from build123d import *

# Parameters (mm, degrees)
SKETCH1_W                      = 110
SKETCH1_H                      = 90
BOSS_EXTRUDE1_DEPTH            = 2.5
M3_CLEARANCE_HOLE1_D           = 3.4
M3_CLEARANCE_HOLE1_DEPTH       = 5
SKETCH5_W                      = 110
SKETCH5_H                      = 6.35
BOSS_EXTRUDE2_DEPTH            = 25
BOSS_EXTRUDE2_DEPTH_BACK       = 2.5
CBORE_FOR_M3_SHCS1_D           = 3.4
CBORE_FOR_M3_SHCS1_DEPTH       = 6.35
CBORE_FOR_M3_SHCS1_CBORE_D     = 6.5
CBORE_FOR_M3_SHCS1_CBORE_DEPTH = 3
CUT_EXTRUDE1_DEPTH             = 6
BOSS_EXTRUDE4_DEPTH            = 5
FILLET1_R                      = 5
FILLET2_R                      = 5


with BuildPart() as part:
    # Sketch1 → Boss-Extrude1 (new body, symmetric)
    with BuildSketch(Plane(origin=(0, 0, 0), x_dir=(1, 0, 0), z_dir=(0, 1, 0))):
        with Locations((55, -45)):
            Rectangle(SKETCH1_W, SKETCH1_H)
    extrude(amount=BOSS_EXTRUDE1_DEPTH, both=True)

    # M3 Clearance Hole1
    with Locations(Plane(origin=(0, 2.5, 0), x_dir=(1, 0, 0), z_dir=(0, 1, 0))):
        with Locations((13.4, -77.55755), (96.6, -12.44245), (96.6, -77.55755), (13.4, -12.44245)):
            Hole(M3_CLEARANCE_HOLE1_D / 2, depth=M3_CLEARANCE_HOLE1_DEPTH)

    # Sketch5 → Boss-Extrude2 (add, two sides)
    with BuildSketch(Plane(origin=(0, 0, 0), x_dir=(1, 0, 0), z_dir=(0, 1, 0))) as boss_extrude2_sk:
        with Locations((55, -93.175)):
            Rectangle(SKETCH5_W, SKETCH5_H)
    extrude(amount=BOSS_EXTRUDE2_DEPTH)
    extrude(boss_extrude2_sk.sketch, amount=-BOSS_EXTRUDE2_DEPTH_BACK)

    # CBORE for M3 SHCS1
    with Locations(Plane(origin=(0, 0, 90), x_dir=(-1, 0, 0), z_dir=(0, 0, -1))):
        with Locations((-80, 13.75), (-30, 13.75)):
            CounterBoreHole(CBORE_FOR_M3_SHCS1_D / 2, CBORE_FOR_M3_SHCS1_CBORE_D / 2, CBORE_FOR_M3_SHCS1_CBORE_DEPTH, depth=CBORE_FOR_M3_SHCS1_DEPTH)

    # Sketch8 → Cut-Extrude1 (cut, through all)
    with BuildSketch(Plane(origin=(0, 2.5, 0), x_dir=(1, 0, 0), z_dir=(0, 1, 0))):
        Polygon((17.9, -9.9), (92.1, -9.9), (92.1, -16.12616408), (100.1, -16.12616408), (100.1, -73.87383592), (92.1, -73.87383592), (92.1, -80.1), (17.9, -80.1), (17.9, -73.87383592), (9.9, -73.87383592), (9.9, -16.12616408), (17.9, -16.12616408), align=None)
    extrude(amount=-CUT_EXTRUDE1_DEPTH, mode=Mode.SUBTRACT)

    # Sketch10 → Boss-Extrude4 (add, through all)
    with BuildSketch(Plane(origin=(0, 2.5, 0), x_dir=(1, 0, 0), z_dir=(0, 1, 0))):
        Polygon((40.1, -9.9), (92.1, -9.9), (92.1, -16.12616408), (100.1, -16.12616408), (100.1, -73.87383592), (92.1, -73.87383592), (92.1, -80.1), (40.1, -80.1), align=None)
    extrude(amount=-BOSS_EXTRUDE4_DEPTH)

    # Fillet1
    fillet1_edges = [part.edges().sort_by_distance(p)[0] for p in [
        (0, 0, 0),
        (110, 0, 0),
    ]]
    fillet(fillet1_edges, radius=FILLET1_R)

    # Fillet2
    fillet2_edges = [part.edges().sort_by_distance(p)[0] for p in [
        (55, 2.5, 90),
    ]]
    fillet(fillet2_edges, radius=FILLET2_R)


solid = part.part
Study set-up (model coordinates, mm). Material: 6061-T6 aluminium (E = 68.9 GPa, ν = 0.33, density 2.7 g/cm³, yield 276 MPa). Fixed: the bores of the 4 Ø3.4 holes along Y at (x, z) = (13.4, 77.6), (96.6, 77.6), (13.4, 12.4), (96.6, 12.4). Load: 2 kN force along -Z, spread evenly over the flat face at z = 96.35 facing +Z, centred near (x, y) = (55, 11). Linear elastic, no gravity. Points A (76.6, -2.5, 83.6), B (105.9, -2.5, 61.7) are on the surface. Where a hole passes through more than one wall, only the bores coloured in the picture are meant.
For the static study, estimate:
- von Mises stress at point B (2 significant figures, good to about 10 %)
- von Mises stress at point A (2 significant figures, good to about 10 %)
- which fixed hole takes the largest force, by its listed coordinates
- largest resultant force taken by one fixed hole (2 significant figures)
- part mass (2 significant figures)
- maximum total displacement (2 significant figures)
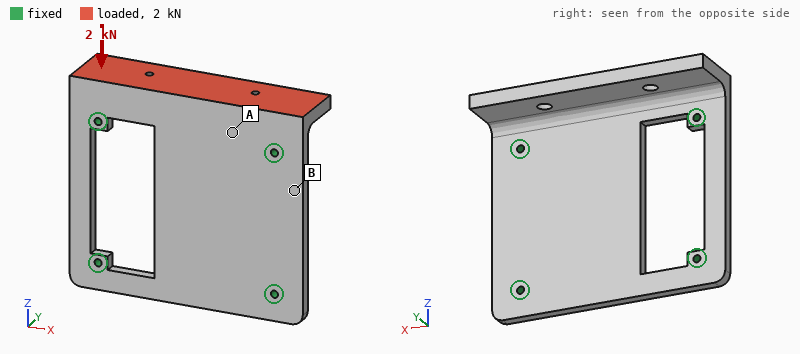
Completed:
11 MPa
38 MPa
(96.6, 77.6)
890 N
160 g
0.20 mm
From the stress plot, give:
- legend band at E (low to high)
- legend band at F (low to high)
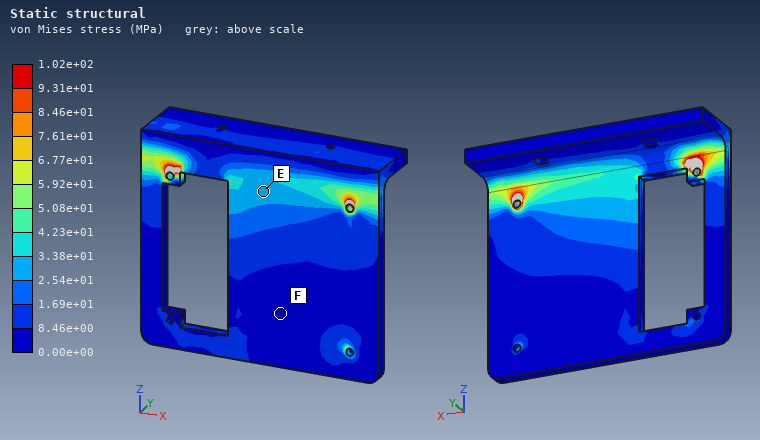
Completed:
2.54e+01 to 3.38e+01 MPa
0.00e+00 to 8.46e+00 MPa
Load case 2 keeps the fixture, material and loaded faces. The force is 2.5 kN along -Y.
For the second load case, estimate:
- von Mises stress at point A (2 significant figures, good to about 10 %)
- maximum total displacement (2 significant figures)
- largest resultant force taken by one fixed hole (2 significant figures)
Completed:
50 MPa
0.31 mm
1.5 kN
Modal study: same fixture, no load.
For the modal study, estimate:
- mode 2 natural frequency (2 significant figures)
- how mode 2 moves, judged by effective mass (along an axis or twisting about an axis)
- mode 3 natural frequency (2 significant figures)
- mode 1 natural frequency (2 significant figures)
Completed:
2600 Hz
along Y
3900 Hz
2100 Hz
